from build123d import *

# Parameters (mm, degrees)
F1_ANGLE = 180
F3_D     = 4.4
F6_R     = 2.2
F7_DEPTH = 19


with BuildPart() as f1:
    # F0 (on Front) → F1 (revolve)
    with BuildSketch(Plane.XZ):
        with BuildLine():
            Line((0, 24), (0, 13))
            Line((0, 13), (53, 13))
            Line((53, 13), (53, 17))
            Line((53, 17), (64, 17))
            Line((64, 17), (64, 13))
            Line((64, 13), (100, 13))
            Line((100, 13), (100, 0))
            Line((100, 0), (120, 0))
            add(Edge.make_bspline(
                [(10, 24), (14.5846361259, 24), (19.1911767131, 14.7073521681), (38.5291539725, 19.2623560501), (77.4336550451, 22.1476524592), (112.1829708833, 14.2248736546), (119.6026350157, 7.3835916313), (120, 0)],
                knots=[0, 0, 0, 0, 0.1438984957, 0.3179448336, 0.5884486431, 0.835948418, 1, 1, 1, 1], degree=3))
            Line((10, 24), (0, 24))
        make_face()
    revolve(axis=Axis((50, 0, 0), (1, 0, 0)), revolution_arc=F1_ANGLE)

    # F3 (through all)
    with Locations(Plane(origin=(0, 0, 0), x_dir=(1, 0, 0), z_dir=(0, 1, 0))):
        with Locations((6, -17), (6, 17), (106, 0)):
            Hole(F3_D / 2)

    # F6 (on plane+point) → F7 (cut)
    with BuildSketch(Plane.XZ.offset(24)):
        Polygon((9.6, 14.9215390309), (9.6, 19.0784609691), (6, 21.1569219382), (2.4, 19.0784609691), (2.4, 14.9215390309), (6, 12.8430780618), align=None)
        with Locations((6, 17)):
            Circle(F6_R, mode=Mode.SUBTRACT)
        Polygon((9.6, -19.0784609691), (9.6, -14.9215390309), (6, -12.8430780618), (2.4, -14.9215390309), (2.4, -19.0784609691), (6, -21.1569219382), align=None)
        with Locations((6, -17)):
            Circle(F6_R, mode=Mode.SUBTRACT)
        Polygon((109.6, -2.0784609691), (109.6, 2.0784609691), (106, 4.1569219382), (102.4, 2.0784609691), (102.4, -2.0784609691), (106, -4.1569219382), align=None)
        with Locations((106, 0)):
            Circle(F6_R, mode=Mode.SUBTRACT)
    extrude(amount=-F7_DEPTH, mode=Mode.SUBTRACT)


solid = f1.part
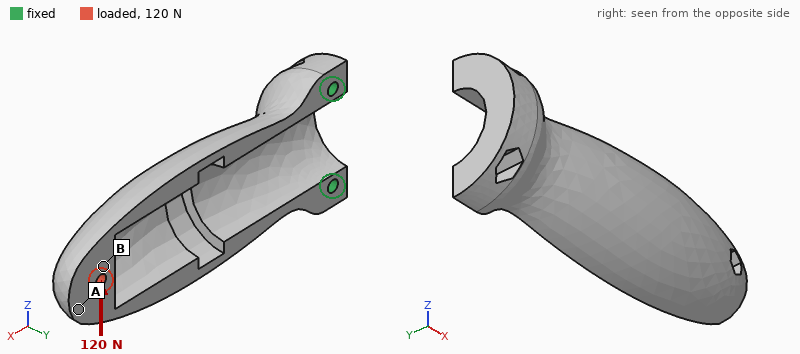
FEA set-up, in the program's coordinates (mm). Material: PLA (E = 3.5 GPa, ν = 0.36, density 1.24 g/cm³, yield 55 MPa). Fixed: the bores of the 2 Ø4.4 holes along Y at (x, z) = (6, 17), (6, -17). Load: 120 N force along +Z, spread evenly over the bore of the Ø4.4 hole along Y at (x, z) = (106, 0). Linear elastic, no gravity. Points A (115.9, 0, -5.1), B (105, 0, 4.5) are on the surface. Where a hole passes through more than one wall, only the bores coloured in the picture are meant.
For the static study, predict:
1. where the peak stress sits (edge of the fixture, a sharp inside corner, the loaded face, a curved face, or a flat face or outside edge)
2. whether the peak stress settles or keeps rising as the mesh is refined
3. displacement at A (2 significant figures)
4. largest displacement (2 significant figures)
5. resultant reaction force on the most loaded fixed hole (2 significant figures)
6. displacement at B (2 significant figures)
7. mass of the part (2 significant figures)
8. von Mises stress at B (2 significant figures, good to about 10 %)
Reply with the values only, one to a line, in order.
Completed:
edge of the fixture
keeps rising
1.5 mm
1.6 mm
310 N
1.4 mm
46 g
3.7 MPa
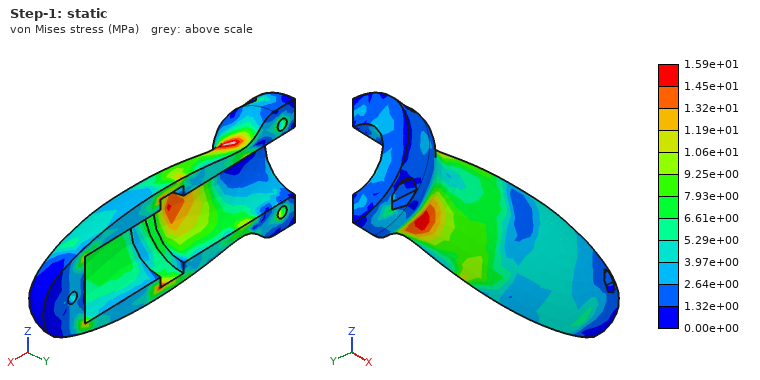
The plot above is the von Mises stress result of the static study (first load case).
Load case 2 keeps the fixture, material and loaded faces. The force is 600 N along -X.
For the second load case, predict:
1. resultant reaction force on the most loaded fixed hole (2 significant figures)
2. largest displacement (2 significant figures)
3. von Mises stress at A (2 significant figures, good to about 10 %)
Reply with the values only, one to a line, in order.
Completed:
300 N
1.5 mm
4.0 MPa
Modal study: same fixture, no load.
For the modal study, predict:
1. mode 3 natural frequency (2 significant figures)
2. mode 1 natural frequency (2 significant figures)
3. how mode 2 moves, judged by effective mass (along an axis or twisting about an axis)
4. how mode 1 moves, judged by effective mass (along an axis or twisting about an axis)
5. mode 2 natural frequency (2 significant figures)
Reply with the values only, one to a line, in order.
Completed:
1100 Hz
230 Hz
along Z
along Y
430 Hz
